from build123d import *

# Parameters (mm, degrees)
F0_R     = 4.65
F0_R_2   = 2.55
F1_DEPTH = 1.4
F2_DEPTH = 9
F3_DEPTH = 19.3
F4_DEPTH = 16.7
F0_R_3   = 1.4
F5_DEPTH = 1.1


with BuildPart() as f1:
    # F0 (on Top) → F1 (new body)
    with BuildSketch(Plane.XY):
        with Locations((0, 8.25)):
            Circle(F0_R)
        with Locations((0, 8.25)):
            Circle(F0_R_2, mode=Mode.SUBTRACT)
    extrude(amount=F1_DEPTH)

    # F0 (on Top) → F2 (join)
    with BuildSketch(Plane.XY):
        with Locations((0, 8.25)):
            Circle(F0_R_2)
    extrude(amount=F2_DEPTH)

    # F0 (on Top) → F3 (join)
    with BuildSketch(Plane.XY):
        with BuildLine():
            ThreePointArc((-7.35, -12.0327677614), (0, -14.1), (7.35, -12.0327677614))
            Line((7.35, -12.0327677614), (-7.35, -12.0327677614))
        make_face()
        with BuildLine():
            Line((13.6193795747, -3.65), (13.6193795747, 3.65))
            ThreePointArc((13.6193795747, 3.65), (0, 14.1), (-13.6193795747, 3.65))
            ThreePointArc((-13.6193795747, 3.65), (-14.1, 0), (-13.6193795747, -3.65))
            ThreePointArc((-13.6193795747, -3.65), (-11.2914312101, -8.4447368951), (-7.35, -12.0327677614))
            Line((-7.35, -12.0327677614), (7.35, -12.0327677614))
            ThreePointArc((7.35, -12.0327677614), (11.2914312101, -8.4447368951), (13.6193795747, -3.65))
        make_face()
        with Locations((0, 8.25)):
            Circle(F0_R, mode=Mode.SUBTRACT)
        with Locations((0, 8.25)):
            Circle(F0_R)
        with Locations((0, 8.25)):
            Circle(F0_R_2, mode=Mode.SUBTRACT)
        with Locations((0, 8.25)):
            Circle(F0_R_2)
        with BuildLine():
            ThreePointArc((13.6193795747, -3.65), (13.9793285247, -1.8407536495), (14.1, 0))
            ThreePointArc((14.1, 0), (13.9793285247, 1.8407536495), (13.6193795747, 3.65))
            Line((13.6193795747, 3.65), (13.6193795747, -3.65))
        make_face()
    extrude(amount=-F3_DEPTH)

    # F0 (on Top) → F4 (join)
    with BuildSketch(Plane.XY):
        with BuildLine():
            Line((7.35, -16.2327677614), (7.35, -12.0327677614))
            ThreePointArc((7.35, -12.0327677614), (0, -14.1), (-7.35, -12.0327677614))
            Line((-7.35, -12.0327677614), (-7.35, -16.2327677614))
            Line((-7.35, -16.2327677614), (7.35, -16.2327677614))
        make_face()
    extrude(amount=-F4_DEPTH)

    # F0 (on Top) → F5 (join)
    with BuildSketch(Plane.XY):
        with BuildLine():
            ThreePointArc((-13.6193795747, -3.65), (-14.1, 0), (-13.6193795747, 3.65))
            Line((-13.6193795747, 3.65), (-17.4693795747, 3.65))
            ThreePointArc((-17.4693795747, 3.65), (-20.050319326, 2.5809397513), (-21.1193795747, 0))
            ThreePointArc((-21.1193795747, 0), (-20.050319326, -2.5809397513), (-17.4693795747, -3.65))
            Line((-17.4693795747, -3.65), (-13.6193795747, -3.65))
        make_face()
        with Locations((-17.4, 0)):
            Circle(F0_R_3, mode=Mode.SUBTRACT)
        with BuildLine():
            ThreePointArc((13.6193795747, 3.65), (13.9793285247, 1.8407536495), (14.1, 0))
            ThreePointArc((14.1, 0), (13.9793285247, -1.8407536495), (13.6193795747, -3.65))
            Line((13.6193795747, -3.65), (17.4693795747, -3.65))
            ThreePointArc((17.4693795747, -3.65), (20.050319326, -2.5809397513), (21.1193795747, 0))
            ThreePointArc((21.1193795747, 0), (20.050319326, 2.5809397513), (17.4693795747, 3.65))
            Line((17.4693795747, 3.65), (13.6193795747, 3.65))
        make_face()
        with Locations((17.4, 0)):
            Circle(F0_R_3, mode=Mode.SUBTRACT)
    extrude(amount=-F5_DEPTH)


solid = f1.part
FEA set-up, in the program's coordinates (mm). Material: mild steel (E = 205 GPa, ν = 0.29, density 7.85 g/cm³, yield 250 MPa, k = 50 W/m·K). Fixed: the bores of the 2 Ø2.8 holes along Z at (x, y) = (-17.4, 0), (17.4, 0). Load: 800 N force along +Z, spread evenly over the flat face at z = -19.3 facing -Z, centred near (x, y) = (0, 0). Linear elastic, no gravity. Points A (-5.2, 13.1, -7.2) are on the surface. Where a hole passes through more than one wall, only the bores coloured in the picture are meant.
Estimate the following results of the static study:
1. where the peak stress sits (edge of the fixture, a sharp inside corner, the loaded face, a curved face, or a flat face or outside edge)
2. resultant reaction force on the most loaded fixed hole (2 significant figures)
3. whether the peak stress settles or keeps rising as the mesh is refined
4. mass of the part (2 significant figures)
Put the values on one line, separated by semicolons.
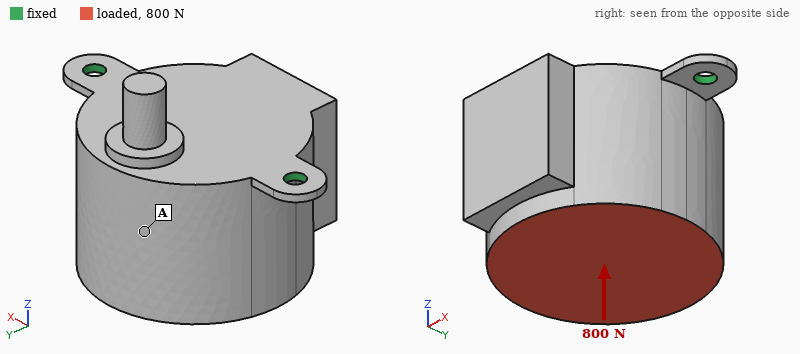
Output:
edge of the fixture; 460 N; keeps rising; 100 g
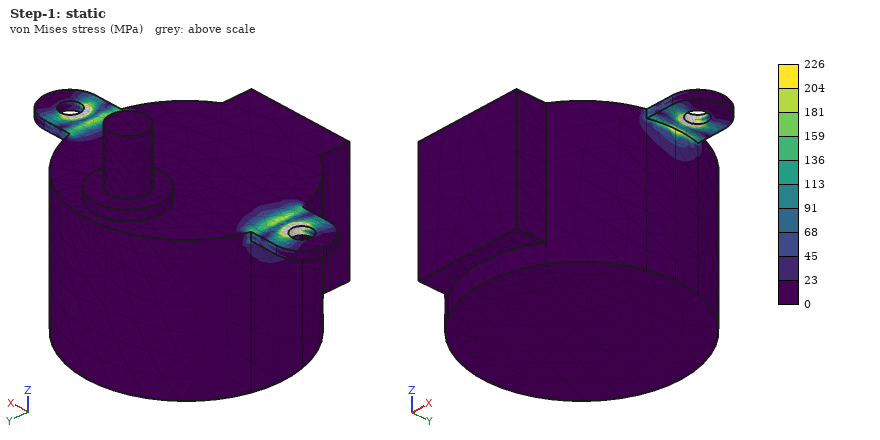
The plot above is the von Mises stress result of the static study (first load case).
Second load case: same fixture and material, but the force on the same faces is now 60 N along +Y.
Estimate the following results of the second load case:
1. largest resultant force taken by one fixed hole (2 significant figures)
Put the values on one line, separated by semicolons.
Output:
30 N
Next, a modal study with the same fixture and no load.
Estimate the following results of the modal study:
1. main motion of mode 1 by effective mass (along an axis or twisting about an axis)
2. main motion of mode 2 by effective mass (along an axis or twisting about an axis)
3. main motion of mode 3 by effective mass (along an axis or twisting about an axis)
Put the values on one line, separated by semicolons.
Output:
along Y; along Z; along X
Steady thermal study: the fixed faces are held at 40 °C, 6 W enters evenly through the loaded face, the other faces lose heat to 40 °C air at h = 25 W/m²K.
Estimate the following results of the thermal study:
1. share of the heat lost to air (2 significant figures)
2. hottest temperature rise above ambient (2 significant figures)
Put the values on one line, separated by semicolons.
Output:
28 %; 27 K
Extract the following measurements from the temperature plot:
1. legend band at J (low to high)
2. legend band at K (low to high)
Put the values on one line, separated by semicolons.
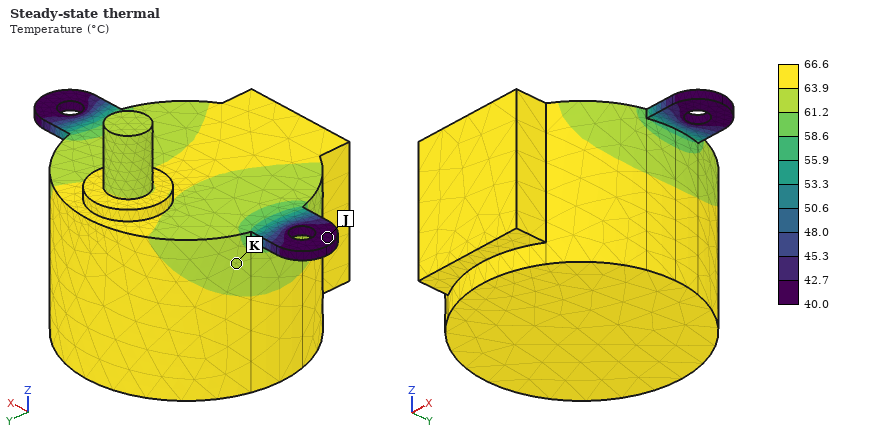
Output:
40.0 to 42.7 °C; 61.2 to 63.9 °C
